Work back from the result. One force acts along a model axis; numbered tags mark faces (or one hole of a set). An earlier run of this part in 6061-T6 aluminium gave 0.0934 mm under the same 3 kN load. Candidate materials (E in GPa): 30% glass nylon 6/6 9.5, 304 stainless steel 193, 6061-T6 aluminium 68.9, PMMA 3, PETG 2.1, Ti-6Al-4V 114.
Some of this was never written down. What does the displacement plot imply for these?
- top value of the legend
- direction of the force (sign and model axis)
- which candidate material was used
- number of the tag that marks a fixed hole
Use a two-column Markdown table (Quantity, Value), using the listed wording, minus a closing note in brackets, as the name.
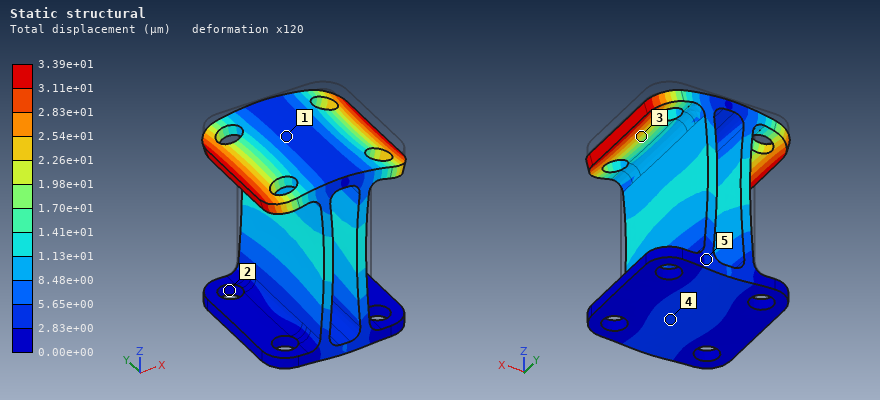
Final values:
| Quantity | Value |
|---|---|
| top value of the legend | 3.39e+01 µm |
| direction of the force | -Z |
| which candidate material was used | 304 stainless steel |
| number of the tag that marks a fixed hole | 2 |
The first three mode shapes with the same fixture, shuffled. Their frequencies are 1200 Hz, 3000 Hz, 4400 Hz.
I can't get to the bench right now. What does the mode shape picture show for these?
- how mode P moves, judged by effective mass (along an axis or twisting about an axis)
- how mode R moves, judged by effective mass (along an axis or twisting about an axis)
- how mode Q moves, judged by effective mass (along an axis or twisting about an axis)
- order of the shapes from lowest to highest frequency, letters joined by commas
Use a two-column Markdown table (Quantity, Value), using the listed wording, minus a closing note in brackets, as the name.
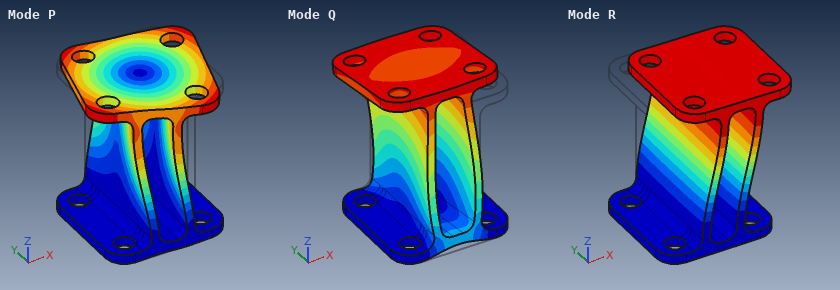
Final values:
| Quantity | Value |
|---|---|
| how mode P moves, judged by effective mass | twisting about Z |
| how mode R moves, judged by effective mass | along X |
| how mode Q moves, judged by effective mass | along Y |
| order of the shapes from lowest to highest frequency, letters joined by commas | R, P, Q |
